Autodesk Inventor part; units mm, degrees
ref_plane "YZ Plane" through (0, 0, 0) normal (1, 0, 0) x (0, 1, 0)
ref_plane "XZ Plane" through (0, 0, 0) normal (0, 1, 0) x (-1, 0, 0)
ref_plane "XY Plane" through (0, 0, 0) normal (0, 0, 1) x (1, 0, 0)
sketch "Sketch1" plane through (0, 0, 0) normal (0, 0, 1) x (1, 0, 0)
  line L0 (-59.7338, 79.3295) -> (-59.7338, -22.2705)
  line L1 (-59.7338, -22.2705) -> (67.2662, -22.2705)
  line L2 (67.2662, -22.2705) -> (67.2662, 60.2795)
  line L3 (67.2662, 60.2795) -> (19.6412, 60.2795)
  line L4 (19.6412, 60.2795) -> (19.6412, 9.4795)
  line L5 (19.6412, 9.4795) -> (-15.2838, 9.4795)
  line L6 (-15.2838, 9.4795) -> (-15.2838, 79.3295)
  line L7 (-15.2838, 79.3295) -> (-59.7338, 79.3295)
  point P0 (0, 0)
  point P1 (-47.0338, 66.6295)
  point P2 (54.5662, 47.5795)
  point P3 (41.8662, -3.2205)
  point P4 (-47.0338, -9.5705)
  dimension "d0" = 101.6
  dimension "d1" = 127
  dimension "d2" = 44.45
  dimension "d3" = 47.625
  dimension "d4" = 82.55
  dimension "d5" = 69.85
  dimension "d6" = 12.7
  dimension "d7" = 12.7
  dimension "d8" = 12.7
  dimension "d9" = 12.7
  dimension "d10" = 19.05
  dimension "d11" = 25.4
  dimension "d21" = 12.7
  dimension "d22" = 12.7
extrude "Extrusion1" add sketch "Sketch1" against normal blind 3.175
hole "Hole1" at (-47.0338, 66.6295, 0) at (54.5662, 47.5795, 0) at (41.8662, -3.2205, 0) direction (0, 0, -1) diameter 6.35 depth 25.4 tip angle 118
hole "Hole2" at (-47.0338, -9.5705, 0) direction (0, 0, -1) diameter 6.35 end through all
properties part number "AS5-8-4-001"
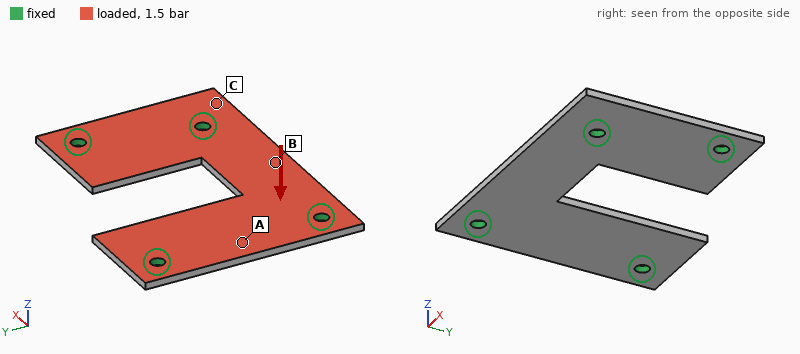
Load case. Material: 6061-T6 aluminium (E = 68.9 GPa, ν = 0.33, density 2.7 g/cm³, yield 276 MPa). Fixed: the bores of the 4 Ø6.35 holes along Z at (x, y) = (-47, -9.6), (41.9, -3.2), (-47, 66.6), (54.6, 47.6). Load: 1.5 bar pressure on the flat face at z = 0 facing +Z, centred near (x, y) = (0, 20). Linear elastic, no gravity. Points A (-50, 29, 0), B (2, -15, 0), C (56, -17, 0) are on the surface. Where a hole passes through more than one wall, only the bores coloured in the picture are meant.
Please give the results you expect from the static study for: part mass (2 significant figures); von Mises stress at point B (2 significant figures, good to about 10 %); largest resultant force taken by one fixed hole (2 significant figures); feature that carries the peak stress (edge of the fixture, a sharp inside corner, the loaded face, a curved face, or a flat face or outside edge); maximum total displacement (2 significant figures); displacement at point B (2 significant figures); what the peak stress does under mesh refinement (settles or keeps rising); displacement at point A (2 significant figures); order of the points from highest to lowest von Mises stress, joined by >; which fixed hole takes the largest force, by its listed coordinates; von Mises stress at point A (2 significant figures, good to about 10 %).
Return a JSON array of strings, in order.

["81 g", "27 MPa", "450 N", "edge of the fixture", "0.21 mm", "0.12 mm", "keeps rising", "0.066 mm", "B > A > C", "(41.9, -3.2)", "21 MPa"]
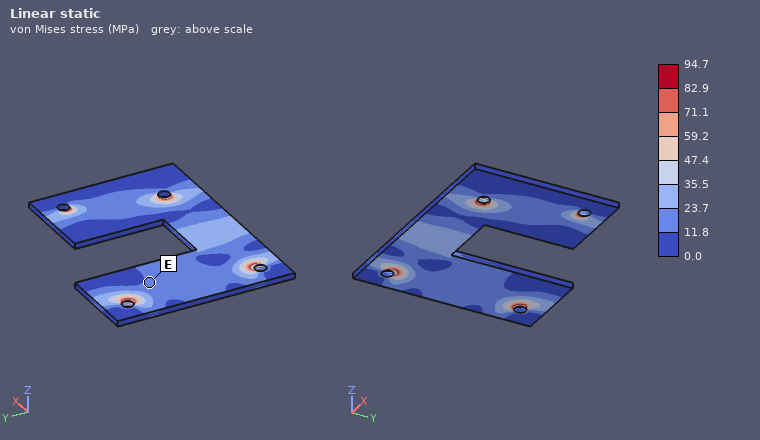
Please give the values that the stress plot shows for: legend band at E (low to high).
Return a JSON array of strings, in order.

["11.8 to 23.7 MPa"]
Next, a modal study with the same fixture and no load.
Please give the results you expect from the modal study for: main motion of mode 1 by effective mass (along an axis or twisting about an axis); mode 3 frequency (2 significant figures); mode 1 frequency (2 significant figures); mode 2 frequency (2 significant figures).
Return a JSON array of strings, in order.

["along Z", "2700 Hz", "2000 Hz", "2500 Hz"]
